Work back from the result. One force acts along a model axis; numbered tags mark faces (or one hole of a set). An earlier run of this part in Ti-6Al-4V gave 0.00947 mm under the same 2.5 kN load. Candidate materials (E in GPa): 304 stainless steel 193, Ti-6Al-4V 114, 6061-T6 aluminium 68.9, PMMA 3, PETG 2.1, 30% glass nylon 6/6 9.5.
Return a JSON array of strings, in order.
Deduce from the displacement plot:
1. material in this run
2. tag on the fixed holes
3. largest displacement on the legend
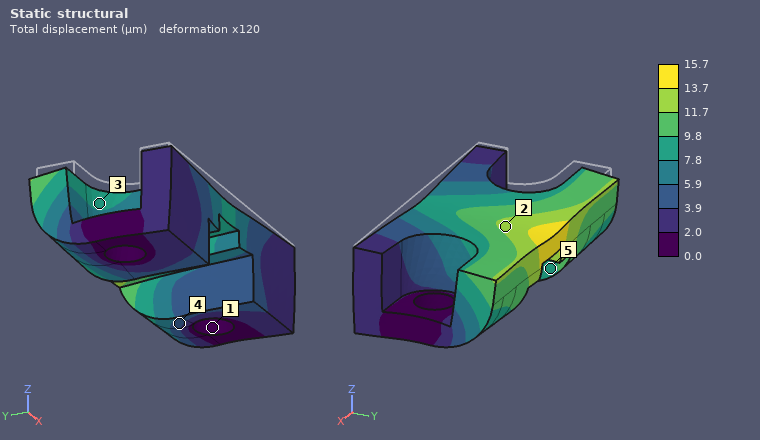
["6061-T6 aluminium", "1", "15.7 µm"]
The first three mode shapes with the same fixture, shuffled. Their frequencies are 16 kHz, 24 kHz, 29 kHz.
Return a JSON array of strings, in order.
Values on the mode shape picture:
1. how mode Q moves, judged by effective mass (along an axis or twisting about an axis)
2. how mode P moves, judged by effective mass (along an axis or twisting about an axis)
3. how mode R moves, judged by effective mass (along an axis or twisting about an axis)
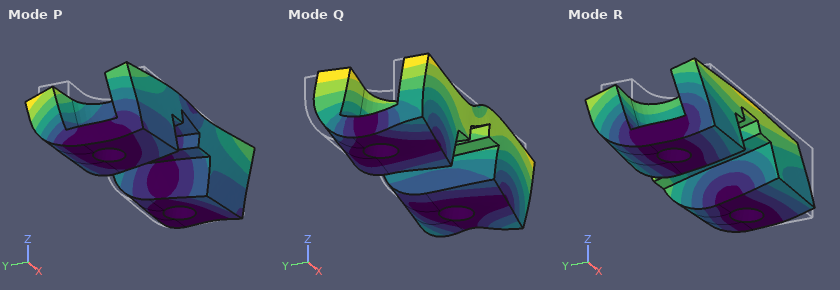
["along X", "twisting about Z", "along Y"]
